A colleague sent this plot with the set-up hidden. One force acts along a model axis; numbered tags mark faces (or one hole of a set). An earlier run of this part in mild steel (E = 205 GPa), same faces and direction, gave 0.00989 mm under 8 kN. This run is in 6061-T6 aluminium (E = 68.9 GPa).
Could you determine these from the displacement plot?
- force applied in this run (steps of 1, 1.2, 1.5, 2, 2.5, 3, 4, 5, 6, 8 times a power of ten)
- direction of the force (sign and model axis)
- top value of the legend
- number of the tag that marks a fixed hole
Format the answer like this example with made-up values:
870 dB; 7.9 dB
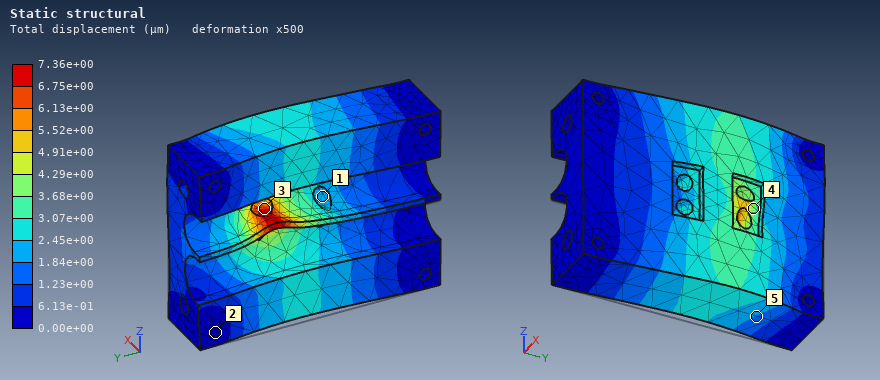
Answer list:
2 kN; +Z; 7.36e+00 µm; 2
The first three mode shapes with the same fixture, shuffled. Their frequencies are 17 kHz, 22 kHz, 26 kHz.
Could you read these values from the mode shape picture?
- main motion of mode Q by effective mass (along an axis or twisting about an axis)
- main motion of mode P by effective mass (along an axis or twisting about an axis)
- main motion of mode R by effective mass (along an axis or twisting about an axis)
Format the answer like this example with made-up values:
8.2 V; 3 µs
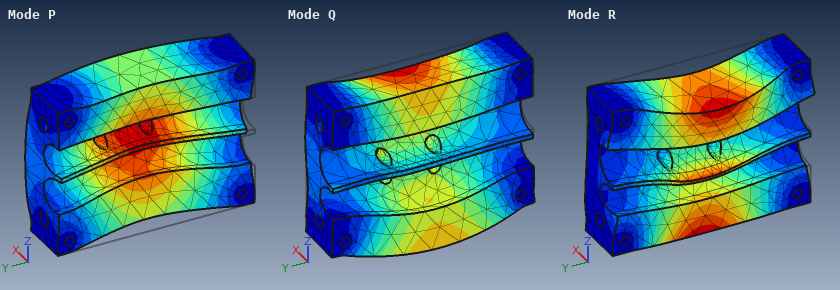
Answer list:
along Z; along X; along Z
